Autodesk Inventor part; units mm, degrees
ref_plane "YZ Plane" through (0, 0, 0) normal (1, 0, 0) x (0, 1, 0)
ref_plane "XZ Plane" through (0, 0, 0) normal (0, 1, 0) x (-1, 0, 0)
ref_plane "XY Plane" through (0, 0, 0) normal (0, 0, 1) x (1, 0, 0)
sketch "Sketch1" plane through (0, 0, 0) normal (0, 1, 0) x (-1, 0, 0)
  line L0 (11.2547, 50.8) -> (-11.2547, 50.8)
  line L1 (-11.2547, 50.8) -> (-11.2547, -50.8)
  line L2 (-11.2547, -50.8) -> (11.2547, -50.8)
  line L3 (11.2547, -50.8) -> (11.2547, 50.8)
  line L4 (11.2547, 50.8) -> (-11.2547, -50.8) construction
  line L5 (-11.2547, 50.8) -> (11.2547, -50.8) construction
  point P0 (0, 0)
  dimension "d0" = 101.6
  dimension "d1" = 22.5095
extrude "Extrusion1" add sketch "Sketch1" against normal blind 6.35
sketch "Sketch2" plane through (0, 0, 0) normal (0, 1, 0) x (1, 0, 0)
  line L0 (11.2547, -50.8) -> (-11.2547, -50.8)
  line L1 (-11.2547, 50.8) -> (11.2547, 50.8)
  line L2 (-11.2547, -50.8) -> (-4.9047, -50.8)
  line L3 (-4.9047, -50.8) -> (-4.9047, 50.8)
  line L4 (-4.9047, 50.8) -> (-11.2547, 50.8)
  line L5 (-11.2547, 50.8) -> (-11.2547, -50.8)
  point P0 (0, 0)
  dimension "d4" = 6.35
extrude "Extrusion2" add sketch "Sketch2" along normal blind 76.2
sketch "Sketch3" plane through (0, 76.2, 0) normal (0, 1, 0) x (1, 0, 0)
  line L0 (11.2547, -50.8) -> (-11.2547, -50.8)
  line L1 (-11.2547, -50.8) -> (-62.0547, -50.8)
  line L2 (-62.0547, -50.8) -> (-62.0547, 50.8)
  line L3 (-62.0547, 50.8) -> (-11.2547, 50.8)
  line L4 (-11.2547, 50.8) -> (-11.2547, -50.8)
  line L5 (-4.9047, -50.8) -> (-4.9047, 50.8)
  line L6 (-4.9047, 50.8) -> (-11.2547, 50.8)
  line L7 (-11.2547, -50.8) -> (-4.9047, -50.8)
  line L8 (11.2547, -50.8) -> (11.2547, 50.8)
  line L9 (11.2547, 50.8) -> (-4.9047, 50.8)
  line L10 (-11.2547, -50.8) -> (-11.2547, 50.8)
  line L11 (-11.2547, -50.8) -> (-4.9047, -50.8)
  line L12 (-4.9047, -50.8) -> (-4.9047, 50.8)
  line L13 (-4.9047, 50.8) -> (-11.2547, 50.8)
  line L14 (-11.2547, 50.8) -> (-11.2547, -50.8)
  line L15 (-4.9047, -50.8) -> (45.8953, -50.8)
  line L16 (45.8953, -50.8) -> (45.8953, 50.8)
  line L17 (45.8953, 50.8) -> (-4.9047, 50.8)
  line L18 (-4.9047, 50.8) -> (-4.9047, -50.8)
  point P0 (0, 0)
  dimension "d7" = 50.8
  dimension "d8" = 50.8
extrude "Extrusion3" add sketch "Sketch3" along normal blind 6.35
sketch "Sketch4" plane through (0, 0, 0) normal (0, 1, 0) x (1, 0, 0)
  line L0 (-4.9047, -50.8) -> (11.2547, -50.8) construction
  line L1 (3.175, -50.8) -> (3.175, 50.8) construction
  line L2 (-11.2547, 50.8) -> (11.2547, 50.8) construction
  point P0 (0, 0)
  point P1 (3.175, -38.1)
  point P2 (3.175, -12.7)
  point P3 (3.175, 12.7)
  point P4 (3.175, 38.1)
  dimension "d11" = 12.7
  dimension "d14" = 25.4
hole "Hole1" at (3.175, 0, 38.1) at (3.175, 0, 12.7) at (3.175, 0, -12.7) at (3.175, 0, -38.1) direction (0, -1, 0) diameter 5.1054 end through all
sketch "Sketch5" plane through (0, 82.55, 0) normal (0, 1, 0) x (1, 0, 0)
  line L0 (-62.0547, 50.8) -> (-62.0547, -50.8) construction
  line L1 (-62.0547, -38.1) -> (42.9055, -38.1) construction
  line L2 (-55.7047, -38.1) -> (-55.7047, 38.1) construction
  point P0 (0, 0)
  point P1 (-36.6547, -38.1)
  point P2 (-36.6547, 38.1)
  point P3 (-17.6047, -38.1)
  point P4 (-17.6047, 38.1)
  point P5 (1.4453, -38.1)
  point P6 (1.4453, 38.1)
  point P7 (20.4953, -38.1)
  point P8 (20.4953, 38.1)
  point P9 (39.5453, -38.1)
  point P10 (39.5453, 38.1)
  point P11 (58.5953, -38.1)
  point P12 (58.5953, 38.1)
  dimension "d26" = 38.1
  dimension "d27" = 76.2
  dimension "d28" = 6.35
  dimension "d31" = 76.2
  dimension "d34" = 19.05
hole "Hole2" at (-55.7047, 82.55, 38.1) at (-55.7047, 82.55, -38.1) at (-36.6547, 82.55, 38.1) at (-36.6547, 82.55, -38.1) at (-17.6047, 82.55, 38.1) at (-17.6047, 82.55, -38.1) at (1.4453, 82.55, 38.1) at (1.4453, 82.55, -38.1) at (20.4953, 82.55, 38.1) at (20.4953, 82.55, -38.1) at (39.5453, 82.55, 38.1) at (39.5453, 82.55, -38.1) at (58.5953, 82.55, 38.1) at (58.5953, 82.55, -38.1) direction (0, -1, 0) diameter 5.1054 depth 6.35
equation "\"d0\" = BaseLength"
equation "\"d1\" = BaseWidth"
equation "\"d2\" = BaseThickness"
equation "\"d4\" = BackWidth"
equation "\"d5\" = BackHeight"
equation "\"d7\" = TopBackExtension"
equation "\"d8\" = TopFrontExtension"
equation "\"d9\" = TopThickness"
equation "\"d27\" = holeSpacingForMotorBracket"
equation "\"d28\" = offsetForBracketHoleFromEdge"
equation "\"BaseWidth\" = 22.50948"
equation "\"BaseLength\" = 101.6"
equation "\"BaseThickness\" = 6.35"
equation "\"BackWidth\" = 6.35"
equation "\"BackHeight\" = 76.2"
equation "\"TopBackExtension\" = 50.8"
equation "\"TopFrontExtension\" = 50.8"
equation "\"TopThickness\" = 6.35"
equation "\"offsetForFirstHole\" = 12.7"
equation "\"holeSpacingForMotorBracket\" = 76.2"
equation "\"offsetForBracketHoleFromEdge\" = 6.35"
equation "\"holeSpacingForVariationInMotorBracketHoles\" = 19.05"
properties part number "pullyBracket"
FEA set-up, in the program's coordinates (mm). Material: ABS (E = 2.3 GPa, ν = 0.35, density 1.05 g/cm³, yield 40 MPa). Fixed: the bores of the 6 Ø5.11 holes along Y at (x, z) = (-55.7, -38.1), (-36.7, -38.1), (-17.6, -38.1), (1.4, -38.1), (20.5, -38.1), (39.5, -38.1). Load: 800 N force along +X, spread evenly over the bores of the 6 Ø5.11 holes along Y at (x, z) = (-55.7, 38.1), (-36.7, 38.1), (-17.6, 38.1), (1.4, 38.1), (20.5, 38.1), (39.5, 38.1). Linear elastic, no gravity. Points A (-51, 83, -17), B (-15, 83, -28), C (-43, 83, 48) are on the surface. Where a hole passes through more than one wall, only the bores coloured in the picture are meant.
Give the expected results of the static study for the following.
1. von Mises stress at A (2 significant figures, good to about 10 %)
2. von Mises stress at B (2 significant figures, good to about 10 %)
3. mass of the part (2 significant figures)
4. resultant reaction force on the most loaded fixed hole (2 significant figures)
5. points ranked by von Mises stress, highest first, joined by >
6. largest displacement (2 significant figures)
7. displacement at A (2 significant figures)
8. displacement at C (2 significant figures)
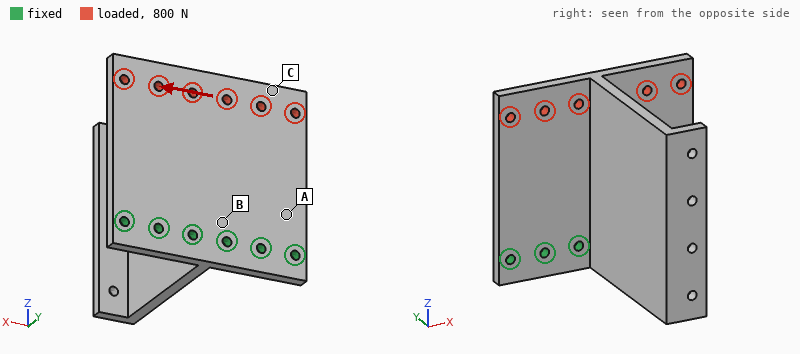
3.2 MPa
2.3 MPa
140 g
490 N
A > B > C
0.25 mm
0.051 mm
0.23 mm
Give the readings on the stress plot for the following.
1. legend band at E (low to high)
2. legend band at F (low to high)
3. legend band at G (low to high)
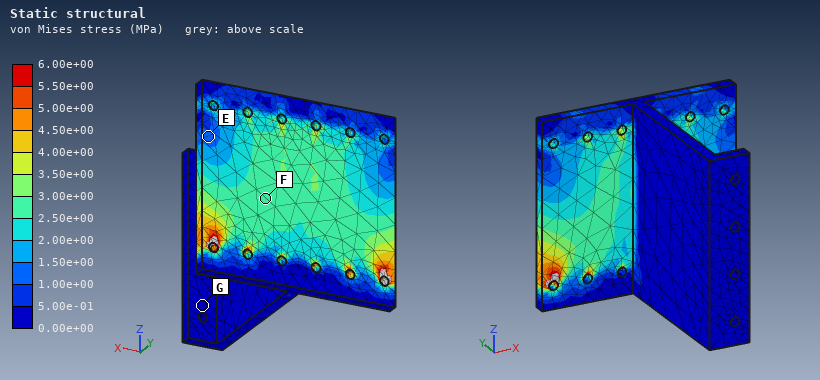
1.00e+00 to 1.50e+00 MPa
2.50e+00 to 3.00e+00 MPa
0.00e+00 to 5.00e-01 MPa
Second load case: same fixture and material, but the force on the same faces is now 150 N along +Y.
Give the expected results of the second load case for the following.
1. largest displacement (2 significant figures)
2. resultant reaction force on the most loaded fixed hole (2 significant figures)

1.9 mm
54 N
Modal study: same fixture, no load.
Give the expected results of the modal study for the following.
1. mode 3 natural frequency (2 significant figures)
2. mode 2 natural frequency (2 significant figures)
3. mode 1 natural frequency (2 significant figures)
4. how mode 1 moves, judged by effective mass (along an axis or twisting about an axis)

340 Hz
190 Hz
140 Hz
along X
